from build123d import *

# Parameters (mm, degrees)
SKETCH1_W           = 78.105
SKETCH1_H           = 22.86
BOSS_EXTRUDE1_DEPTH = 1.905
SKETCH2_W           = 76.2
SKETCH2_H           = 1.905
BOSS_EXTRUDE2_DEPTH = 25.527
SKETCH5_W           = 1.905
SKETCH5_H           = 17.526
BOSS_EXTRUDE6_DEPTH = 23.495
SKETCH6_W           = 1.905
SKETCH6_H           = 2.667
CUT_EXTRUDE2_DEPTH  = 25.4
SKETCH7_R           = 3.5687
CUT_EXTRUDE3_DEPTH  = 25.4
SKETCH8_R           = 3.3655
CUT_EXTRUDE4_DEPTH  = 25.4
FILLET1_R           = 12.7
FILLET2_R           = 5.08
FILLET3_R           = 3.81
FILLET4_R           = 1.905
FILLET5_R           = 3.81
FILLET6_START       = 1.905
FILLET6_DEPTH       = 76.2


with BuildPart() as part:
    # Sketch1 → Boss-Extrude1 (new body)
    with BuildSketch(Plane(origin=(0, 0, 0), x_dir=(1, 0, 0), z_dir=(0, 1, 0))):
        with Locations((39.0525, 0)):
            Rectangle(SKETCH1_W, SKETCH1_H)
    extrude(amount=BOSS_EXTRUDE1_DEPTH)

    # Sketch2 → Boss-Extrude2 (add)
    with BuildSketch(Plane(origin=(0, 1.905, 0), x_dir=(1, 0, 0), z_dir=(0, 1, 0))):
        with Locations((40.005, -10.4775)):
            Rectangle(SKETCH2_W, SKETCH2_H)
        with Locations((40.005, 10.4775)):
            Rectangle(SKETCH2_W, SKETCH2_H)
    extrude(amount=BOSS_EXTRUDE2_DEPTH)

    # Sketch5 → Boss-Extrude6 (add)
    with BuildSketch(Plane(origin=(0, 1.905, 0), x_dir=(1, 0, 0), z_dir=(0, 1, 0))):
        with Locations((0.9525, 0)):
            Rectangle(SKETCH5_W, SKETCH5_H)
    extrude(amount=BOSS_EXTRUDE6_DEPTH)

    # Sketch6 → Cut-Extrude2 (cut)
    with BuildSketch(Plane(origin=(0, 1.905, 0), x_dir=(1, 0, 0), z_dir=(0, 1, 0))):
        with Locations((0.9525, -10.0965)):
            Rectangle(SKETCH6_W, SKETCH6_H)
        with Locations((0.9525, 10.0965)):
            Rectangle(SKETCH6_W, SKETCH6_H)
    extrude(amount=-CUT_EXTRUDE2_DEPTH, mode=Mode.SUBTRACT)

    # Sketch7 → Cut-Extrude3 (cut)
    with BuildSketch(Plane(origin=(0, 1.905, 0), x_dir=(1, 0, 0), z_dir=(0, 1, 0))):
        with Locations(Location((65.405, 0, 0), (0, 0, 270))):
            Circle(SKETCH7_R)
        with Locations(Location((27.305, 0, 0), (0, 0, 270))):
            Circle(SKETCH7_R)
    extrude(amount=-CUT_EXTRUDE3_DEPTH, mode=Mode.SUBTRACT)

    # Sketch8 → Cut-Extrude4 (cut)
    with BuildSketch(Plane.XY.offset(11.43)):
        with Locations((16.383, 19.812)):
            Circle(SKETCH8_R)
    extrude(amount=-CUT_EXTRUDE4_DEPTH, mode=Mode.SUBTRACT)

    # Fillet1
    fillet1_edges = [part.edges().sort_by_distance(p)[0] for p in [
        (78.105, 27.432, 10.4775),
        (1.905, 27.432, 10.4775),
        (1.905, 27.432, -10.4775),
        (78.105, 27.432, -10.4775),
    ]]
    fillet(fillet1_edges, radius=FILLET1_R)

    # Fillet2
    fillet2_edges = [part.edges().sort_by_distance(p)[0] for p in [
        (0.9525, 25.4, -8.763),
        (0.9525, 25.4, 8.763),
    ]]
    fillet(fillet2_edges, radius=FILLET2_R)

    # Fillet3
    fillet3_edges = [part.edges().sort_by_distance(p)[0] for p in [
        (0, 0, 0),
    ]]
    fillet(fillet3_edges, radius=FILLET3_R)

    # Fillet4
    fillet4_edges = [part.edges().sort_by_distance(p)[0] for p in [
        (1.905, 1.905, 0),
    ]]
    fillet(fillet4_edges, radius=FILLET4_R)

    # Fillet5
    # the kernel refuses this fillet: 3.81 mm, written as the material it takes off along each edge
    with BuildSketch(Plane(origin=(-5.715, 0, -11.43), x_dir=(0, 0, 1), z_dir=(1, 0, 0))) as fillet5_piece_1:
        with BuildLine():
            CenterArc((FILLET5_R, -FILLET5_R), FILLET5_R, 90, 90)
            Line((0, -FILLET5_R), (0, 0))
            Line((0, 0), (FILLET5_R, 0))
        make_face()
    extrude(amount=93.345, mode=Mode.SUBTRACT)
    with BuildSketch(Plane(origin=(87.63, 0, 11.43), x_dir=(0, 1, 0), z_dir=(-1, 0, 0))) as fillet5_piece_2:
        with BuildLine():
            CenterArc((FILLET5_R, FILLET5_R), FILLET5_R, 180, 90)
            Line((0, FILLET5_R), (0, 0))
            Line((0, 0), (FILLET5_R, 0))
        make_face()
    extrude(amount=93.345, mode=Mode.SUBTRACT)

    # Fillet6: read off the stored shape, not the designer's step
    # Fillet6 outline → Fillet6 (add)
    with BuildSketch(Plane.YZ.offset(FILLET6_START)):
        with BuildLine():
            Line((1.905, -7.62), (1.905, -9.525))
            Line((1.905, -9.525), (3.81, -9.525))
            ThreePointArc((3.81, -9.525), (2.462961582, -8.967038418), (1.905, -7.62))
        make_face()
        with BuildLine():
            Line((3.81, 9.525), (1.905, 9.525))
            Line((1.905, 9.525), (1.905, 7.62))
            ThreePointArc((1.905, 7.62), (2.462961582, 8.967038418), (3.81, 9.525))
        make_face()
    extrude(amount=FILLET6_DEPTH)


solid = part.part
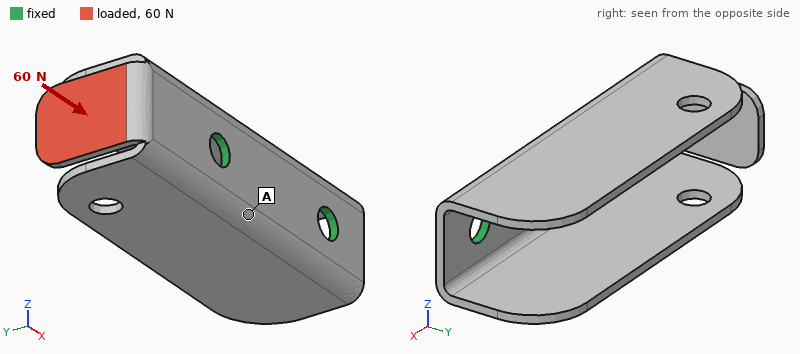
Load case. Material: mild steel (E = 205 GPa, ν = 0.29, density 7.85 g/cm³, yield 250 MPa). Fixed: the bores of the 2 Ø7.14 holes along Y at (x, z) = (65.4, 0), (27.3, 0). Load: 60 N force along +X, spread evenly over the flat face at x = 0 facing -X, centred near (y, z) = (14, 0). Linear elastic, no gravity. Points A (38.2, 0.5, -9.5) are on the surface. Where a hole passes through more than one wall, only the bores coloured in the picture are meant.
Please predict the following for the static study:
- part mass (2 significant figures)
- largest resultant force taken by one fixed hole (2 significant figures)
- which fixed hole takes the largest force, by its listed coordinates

83 g
39 N
(27.3, 0)
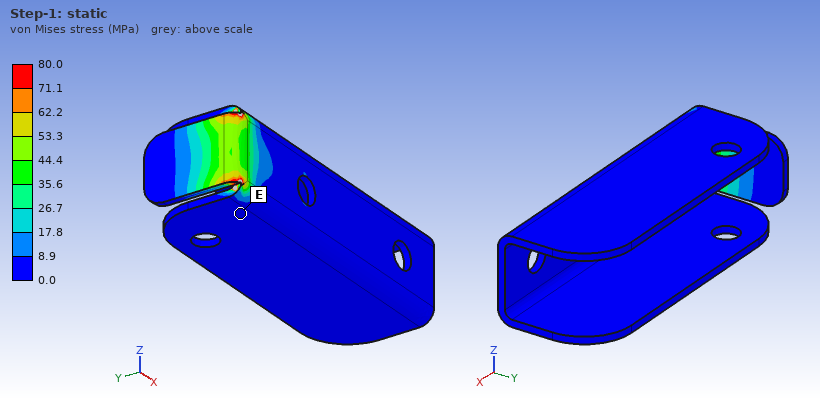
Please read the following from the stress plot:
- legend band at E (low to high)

0.0 to 8.9 MPa
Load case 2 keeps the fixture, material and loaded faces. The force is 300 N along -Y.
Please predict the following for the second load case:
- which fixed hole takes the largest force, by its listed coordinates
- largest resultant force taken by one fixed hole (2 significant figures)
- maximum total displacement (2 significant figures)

(27.3, 0)
510 N
0.10 mm
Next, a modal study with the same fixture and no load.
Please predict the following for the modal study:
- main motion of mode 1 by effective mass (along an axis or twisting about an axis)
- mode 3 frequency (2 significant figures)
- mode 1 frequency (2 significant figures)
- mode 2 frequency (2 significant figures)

along Z
2200 Hz
1500 Hz
1700 Hz
